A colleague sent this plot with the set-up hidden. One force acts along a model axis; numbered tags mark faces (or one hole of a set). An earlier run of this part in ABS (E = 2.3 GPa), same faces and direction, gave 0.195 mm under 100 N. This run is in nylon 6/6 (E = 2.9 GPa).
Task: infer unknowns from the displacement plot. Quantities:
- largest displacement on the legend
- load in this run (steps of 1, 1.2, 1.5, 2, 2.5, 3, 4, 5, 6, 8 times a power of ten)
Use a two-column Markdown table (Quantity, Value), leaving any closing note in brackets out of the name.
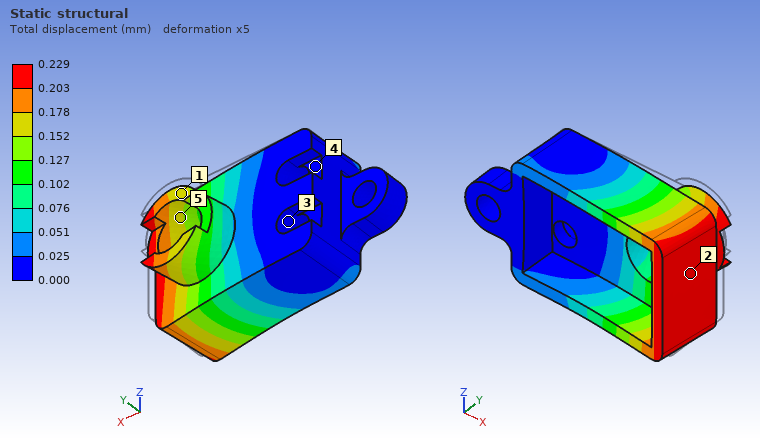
| Quantity | Value |
|---|---|
| largest displacement on the legend | 0.229 mm |
| load in this run | 150 N |
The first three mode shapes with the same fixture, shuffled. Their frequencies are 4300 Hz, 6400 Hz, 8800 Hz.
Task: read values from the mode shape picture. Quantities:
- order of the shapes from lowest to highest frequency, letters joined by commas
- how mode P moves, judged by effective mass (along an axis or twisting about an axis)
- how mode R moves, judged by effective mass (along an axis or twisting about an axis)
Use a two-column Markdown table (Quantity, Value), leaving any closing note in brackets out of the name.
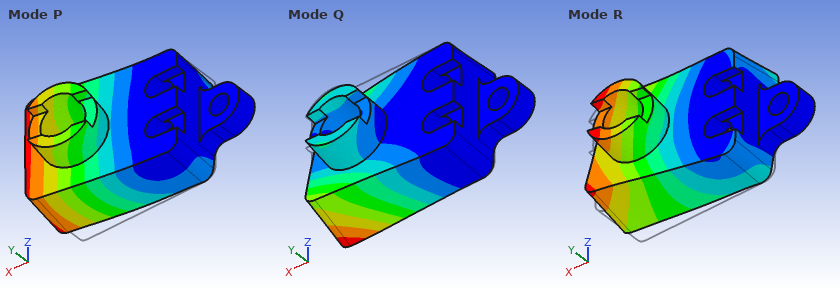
| Quantity | Value |
|---|---|
| order of the shapes from lowest to highest frequency, letters joined by commas | P, Q, R |
| how mode P moves, judged by effective mass | along Y |
| how mode R moves, judged by effective mass | along Z |
